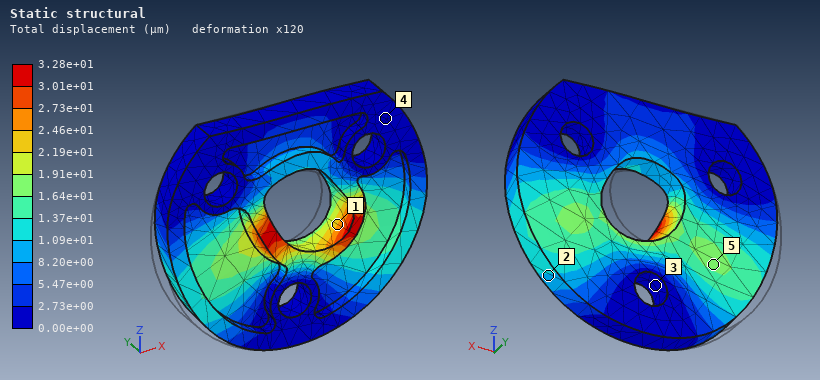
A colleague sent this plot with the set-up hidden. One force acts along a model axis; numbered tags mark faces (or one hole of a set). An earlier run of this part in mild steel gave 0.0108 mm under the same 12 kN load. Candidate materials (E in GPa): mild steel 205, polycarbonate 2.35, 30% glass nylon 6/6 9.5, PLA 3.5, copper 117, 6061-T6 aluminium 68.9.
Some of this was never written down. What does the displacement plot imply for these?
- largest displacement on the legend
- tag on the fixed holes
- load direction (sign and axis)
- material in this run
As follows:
3.28e+01 µm
3
+X
6061-T6 aluminium
